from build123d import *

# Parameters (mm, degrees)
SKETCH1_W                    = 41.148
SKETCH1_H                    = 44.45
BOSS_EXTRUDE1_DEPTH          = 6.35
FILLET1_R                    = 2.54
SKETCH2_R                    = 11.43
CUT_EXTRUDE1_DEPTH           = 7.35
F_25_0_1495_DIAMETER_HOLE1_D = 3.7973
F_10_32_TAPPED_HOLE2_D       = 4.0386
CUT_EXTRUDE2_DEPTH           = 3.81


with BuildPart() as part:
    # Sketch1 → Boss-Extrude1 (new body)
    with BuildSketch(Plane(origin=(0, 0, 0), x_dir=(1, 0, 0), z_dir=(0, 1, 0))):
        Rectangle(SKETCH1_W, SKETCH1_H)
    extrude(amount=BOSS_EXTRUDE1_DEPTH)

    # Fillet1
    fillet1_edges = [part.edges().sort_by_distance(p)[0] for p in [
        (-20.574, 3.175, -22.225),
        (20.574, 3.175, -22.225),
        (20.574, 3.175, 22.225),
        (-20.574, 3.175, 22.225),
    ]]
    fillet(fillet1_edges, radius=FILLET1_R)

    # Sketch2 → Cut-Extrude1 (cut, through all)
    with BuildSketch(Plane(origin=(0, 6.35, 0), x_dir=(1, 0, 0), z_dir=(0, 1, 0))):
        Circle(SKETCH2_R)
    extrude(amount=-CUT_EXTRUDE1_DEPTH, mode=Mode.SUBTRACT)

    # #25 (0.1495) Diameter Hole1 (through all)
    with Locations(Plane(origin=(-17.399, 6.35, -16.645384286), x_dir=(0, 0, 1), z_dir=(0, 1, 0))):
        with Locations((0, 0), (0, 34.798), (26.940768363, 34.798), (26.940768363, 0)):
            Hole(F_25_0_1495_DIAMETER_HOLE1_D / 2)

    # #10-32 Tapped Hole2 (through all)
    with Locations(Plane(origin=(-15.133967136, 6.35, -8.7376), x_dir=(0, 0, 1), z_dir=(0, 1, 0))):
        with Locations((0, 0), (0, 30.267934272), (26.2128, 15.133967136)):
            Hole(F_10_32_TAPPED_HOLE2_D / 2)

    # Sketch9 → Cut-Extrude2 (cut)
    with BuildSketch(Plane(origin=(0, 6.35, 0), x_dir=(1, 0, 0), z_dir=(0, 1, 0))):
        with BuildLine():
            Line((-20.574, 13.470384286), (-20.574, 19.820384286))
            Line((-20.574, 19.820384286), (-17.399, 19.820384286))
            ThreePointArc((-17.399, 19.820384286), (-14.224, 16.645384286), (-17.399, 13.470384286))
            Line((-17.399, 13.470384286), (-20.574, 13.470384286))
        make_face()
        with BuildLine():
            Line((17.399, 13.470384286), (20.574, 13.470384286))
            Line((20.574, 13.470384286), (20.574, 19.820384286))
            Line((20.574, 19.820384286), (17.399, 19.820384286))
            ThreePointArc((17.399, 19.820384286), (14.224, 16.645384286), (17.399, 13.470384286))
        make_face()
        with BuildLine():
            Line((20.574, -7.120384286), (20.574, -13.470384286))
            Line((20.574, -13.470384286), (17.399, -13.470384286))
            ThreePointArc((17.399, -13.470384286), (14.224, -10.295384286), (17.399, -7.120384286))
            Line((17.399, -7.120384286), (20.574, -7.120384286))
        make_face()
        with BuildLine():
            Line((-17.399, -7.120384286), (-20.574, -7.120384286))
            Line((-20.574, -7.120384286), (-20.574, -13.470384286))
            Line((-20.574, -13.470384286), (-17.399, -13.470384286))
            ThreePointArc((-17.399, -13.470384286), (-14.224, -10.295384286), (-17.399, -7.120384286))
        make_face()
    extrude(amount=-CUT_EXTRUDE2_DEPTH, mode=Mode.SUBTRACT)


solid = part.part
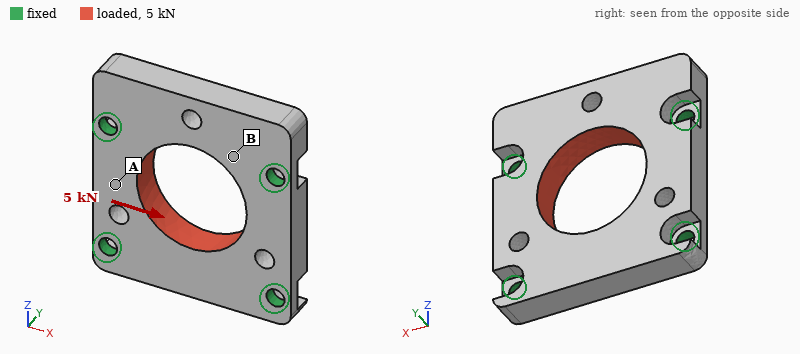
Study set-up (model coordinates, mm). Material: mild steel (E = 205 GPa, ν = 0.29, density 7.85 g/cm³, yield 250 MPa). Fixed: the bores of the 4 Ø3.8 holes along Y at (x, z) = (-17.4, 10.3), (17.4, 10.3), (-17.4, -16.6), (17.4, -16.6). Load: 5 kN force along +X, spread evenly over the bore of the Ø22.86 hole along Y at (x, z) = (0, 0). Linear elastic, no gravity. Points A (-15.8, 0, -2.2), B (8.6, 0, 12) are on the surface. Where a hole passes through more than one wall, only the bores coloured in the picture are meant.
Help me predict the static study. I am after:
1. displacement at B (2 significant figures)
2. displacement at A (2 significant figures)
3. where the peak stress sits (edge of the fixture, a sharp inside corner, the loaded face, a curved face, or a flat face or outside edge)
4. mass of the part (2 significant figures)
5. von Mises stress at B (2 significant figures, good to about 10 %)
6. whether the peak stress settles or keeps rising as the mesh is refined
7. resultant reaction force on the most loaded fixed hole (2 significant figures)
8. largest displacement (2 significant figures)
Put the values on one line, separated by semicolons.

1.5 µm; 2.5 µm; edge of the fixture; 63 g; 32 MPa; keeps rising; 1.4 kN; 3.8 µm
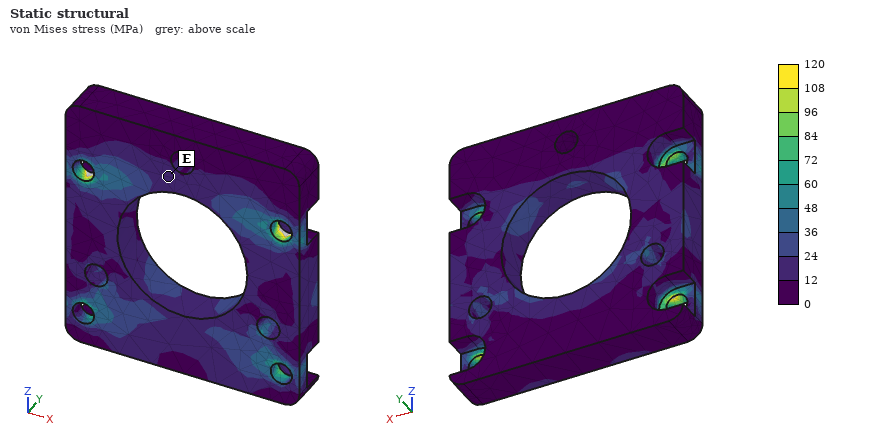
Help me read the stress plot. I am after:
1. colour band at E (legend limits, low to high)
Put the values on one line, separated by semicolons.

12 to 24 MPa
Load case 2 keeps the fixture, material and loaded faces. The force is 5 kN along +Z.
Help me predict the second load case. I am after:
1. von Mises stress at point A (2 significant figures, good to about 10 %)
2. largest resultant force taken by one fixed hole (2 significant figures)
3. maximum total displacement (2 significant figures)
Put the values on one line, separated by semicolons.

23 MPa; 1.5 kN; 5.5 µm
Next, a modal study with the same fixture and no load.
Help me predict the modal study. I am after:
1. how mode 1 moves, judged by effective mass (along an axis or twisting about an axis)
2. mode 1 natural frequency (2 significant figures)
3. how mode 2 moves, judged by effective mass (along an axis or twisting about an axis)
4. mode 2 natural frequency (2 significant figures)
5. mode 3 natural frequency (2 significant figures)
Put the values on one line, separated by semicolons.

along Y; 12 kHz; along Y; 18 kHz; 23 kHz
